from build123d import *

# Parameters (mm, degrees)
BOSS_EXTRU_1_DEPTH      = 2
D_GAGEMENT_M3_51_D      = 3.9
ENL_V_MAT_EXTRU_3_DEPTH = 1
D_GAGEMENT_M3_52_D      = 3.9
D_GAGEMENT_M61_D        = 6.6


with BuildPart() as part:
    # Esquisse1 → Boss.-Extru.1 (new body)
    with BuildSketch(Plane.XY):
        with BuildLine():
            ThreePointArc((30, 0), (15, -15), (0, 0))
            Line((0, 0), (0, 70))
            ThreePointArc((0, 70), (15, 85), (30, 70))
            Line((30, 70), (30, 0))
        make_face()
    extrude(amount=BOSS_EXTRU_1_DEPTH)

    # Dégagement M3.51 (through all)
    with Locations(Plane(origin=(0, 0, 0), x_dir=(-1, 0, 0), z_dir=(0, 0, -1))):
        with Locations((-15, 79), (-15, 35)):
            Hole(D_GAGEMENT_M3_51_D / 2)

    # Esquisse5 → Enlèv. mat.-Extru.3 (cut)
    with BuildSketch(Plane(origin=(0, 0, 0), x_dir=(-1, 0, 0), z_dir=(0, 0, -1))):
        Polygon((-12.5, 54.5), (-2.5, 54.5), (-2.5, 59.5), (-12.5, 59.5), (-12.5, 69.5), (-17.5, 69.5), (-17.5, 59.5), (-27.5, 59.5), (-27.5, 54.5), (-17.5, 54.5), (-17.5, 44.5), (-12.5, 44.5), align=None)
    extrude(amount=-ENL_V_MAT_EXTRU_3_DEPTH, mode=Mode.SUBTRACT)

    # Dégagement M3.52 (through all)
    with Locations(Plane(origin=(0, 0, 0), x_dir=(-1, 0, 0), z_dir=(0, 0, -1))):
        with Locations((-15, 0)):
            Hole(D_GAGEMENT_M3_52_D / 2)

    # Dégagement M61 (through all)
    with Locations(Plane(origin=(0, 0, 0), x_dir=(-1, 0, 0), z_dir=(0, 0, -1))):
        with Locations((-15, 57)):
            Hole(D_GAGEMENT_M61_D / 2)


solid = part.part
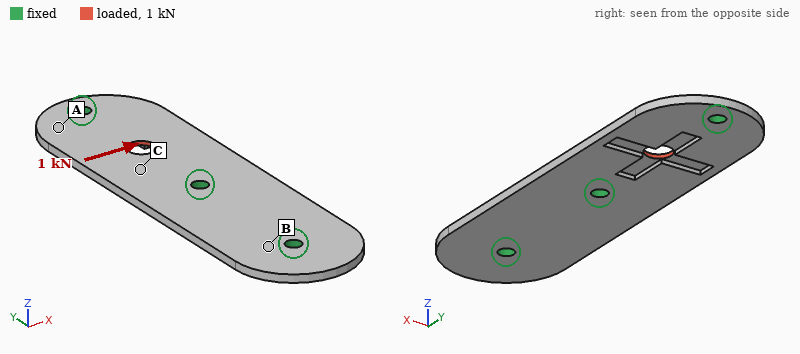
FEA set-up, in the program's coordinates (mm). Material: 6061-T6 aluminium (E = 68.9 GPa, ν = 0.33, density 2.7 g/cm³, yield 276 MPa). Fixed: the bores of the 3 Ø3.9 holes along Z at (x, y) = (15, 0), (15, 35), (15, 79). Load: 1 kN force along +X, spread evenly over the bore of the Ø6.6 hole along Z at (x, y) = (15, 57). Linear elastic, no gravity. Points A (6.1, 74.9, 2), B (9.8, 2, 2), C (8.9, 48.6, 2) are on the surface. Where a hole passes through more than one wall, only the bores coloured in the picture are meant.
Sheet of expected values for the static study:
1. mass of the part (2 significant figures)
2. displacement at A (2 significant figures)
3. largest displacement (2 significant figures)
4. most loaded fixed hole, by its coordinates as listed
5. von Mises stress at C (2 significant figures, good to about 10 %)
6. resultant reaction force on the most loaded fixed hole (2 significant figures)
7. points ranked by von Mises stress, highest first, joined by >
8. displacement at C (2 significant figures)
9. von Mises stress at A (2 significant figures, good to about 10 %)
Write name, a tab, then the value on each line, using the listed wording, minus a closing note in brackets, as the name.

mass of the part	14 g
displacement at A	8.4 µm
largest displacement	34 µm
most loaded fixed hole, by its coordinates as listed	(15, 35)
von Mises stress at C	30 MPa
resultant reaction force on the most loaded fixed hole	630 N
points ranked by von Mises stress, highest first, joined by >	C > A > B
displacement at C	14 µm
von Mises stress at A	16 MPa
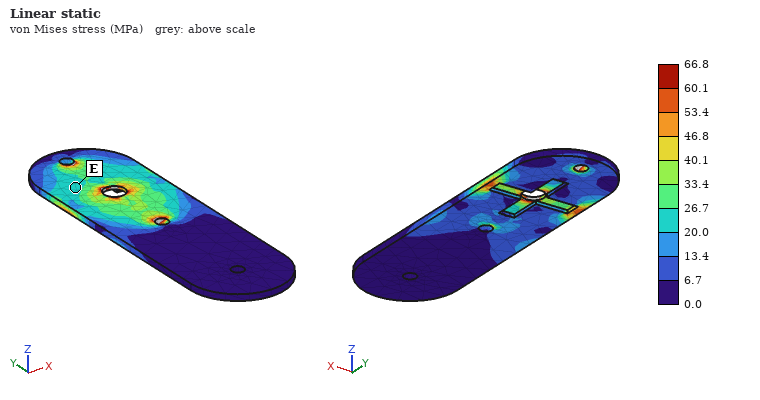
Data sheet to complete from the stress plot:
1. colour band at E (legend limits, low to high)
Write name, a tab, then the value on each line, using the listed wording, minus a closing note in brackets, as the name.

colour band at E	20.0 to 26.7 MPa
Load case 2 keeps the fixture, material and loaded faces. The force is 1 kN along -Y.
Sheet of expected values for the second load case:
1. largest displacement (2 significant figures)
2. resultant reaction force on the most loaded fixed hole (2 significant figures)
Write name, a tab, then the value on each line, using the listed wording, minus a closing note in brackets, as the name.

largest displacement	7.9 µm
resultant reaction force on the most loaded fixed hole	460 N
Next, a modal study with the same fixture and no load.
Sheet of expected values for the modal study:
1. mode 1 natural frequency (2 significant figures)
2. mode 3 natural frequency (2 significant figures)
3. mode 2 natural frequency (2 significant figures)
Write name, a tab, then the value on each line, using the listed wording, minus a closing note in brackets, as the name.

mode 1 natural frequency	4500 Hz
mode 3 natural frequency	5800 Hz
mode 2 natural frequency	4500 Hz
